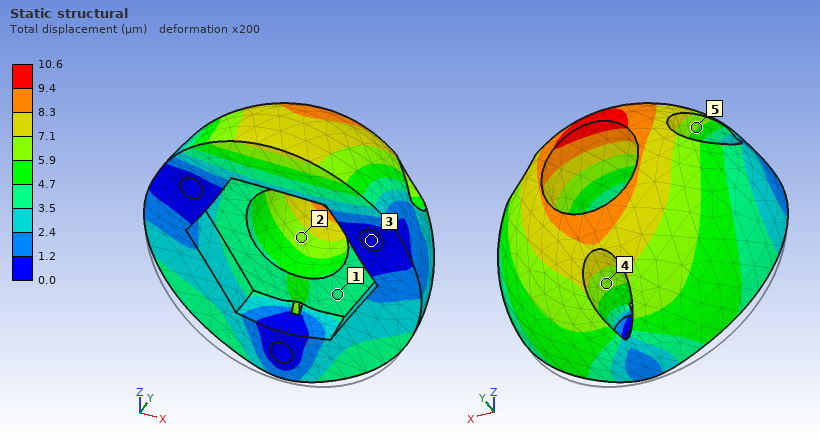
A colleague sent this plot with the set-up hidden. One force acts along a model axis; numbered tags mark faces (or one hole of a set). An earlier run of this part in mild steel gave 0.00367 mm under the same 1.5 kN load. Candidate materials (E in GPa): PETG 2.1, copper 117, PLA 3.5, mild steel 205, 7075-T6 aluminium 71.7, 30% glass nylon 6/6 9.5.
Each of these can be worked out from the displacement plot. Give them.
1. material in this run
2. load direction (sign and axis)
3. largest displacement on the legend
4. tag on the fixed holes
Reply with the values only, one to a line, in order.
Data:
7075-T6 aluminium
+Z
10.6 µm
3
